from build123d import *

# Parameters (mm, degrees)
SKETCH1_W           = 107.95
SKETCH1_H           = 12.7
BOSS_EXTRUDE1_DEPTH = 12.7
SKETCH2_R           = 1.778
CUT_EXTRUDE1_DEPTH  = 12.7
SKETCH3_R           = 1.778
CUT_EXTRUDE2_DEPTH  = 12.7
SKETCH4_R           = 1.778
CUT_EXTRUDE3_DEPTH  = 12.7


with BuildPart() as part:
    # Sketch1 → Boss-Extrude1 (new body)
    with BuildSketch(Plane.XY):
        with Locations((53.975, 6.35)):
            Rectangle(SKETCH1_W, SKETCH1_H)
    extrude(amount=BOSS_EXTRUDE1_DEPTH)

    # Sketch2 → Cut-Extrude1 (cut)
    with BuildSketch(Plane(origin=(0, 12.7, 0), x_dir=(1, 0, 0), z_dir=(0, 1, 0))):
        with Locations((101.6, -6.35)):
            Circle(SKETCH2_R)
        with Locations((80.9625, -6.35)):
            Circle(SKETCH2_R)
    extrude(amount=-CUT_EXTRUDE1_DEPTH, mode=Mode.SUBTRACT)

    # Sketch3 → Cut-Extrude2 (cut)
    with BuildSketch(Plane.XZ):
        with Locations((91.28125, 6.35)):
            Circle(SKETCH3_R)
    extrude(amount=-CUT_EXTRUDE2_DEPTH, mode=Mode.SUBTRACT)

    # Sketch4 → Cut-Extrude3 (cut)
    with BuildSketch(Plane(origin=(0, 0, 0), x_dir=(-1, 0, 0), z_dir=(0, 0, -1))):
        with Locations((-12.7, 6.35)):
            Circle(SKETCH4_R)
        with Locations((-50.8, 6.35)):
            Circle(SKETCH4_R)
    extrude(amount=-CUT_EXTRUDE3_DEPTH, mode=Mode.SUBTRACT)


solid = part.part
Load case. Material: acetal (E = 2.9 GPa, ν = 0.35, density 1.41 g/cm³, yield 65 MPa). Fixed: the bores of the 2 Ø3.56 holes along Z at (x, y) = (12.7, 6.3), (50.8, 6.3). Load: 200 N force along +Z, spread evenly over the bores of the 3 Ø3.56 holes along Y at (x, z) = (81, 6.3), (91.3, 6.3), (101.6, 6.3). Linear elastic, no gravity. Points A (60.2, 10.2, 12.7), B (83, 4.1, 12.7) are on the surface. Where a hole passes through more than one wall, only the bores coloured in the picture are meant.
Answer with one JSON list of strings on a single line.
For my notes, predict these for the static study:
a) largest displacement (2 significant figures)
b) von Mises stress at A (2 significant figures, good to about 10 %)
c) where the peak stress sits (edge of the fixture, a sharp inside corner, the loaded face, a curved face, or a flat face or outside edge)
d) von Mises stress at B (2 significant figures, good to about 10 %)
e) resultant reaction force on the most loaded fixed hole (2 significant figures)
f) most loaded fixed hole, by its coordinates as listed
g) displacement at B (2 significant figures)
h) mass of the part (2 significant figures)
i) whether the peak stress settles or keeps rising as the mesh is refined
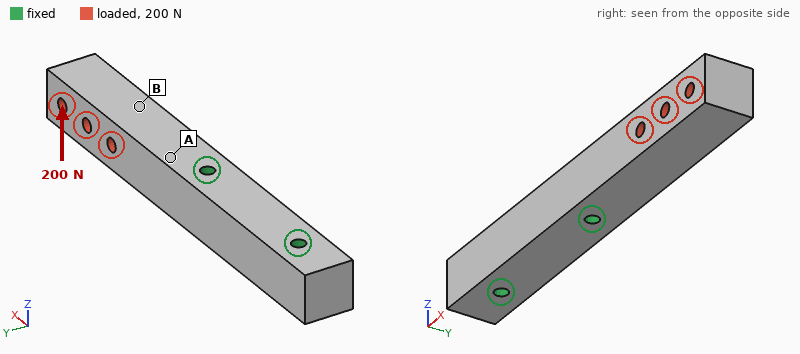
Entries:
["1.3 mm", "18 MPa", "edge of the fixture", "4.5 MPa", "230 N", "(50.8, 6.3)", "0.58 mm", "24 g", "keeps rising"]
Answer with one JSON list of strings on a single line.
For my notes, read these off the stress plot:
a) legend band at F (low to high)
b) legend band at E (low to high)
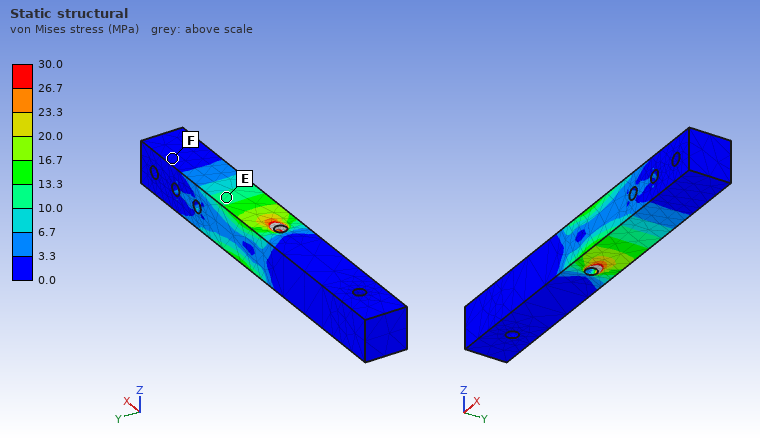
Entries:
["0.0 to 3.3 MPa", "10.0 to 13.3 MPa"]
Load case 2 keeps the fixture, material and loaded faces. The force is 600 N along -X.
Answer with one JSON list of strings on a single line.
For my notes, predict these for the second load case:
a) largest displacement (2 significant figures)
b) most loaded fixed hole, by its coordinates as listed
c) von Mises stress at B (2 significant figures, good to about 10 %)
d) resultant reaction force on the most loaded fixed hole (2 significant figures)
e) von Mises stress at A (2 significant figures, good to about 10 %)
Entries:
["60 µm", "(50.8, 6.3)", "3.4 MPa", "570 N", "3.6 MPa"]
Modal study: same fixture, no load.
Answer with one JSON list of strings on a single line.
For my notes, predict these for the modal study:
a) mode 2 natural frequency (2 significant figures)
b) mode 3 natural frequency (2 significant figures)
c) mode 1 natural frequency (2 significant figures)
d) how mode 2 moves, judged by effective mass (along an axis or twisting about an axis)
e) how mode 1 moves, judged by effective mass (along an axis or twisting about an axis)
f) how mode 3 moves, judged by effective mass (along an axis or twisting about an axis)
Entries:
["880 Hz", "3500 Hz", "770 Hz", "along Z", "along Y", "twisting about X"]
